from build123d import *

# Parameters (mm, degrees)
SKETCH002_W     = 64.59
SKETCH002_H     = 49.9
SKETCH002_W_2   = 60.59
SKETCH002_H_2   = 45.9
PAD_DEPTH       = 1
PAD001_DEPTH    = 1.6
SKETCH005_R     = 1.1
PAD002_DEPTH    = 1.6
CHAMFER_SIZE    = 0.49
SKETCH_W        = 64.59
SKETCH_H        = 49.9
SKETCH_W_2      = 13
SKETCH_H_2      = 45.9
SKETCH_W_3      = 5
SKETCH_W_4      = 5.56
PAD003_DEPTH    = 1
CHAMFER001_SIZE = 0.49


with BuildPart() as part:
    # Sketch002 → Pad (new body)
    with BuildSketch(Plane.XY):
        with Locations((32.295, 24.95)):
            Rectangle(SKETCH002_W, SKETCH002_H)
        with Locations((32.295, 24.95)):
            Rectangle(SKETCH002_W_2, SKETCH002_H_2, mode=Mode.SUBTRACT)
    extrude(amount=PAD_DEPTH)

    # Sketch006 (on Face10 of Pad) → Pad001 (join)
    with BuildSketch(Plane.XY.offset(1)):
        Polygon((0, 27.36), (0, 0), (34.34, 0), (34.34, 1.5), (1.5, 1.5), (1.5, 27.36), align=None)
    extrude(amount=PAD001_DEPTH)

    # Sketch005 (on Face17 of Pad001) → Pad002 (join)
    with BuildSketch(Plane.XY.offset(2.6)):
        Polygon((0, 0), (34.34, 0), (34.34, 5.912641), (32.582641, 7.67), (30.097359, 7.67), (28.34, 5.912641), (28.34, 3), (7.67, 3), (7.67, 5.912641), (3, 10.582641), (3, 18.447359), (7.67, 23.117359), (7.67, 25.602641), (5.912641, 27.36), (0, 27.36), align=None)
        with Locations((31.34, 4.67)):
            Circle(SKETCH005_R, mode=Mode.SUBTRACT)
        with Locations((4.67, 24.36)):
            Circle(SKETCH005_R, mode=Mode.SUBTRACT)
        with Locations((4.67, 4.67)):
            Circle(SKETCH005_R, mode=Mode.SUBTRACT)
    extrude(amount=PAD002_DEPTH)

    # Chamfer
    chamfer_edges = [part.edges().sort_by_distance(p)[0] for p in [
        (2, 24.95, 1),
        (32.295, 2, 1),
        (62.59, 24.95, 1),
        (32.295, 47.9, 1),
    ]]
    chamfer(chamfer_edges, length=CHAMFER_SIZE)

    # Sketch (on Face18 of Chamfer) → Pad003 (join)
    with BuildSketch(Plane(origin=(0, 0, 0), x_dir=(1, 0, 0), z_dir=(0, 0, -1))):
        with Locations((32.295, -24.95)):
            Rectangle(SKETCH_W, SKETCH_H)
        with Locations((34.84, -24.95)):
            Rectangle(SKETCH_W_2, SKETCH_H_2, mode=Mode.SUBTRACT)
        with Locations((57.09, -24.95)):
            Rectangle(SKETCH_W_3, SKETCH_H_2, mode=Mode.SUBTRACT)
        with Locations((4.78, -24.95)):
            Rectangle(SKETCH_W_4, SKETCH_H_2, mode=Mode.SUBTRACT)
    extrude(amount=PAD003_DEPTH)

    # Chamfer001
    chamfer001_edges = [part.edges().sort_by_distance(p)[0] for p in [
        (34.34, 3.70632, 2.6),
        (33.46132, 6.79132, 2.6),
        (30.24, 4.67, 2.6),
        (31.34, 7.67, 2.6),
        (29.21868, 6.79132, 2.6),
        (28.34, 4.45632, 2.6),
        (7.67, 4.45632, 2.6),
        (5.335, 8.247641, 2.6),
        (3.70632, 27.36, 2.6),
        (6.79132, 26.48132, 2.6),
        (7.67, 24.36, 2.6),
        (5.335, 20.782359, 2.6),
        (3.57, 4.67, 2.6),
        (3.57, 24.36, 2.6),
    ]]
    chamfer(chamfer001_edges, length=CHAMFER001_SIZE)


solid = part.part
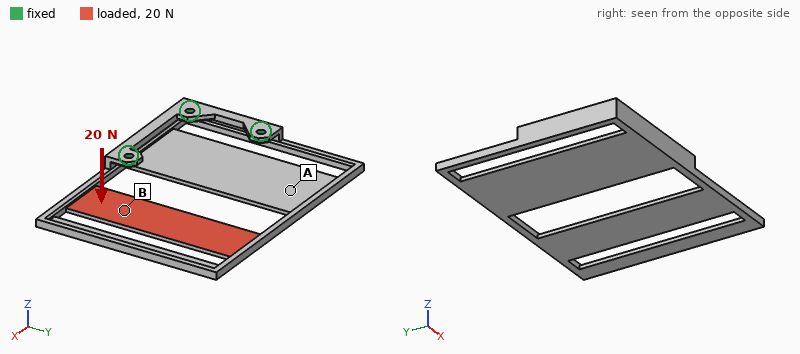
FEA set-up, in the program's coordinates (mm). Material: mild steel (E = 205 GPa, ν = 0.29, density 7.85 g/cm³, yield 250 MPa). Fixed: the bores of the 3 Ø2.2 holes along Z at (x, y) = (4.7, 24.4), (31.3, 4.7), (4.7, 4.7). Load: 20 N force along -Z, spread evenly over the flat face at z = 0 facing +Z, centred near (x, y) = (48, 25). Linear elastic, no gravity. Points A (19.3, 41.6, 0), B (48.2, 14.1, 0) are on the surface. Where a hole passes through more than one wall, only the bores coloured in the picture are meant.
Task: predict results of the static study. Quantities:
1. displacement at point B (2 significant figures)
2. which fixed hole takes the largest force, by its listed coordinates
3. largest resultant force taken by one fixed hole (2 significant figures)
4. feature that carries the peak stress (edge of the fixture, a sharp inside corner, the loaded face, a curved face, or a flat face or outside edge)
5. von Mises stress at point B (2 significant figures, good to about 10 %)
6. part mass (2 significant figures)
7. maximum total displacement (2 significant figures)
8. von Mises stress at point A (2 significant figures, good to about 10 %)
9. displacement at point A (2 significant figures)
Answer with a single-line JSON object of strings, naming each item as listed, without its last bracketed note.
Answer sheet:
{"displacement at point B": "0.26 mm", "which fixed hole takes the largest force, by its listed coordinates": "(31.3, 4.7)", "largest resultant force taken by one fixed hole": "34 N", "feature that carries the peak stress": "a flat face or outside edge", "von Mises stress at point B": "14 MPa", "part mass": "24 g", "maximum total displacement": "0.90 mm", "von Mises stress at point A": "34 MPa", "displacement at point A": "0.22 mm"}
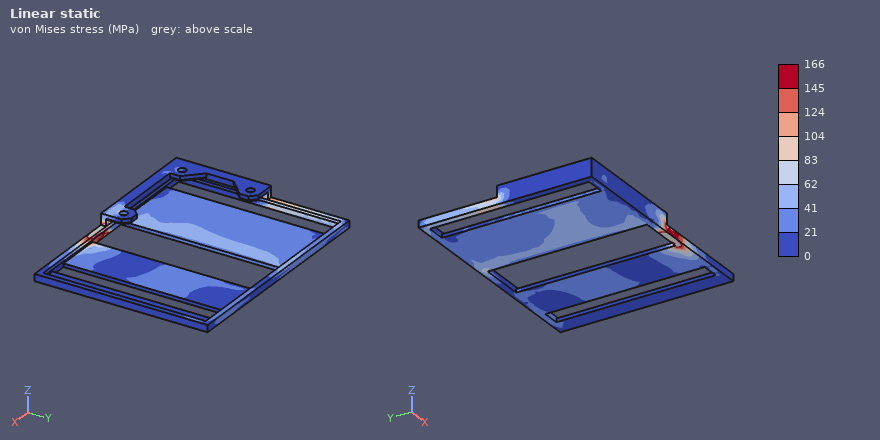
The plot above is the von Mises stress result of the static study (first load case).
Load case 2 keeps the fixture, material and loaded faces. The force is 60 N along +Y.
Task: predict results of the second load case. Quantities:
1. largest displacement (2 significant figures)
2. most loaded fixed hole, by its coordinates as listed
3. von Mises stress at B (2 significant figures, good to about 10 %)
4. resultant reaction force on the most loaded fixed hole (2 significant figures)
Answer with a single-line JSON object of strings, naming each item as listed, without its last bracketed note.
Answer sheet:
{"largest displacement": "51 µm", "most loaded fixed hole, by its coordinates as listed": "(31.3, 4.7)", "von Mises stress at B": "9.0 MPa", "resultant reaction force on the most loaded fixed hole": "88 N"}
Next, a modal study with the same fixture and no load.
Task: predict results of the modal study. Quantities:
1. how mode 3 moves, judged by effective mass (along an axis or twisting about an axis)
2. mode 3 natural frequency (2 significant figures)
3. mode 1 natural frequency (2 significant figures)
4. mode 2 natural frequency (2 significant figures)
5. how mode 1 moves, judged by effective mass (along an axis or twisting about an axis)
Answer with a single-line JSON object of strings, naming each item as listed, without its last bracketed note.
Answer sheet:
{"how mode 3 moves, judged by effective mass": "along Z", "mode 3 natural frequency": "1300 Hz", "mode 1 natural frequency": "280 Hz", "mode 2 natural frequency": "770 Hz", "how mode 1 moves, judged by effective mass": "along Z"}
